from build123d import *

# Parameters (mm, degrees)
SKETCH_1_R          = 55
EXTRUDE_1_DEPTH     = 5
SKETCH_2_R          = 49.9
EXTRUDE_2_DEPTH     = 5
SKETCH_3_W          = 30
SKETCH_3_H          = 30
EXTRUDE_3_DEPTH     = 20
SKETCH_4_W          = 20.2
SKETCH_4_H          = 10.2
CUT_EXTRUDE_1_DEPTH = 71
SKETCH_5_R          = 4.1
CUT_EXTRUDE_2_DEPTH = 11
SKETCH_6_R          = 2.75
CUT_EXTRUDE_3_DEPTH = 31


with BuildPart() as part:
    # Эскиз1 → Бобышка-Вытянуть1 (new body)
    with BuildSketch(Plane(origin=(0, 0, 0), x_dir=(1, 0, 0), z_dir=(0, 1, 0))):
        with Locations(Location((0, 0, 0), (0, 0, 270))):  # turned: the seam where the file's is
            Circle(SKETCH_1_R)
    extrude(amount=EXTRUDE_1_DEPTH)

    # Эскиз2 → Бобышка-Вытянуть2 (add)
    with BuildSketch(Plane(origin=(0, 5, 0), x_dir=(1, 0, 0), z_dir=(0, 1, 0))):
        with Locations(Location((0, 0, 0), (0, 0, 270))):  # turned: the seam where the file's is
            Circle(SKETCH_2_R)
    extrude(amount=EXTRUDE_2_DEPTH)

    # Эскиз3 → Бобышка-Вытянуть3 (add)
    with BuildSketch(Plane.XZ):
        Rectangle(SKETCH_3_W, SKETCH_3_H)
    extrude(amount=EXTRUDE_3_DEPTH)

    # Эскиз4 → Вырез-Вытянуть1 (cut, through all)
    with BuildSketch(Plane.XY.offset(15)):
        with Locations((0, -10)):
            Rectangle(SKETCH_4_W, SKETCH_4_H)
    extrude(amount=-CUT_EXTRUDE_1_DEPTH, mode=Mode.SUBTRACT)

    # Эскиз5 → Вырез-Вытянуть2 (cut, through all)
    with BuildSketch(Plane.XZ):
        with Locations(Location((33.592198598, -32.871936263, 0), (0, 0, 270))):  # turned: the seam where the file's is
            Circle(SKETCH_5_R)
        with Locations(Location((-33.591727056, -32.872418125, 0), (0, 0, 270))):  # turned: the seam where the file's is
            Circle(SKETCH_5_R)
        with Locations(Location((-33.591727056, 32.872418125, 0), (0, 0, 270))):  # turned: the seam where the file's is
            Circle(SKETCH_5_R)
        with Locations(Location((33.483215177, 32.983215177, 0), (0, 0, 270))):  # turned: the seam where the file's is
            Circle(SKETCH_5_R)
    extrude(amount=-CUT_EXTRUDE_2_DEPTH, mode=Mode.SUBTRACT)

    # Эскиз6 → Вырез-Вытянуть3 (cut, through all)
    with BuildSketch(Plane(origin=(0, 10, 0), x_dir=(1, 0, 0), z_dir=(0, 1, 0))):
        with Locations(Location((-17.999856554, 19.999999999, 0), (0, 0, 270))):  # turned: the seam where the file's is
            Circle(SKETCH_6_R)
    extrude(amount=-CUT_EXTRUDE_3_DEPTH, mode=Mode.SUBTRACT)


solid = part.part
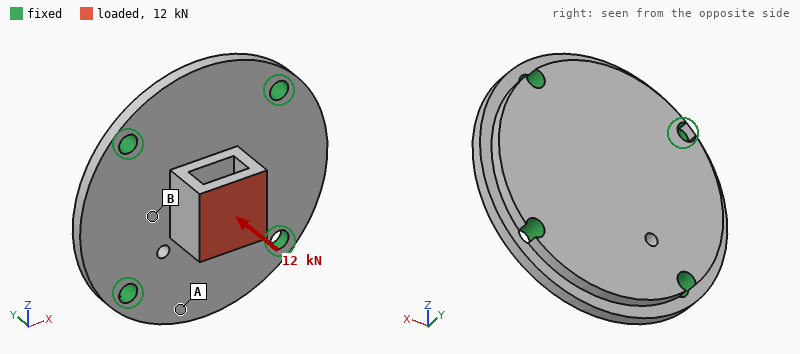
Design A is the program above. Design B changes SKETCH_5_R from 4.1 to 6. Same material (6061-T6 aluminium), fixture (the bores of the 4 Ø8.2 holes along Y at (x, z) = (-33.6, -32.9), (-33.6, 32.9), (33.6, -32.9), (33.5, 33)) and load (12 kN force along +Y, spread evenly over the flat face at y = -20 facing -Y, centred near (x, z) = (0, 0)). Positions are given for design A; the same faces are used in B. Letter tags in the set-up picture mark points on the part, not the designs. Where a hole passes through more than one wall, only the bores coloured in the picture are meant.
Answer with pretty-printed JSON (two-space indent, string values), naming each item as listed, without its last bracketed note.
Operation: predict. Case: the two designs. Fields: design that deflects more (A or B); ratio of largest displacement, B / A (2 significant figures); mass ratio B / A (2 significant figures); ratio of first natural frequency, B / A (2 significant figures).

{
  "design that deflects more": "A",
  "ratio of largest displacement, B / A": "0.90",
  "mass ratio B / A": "0.98",
  "ratio of first natural frequency, B / A": "1.1"
}
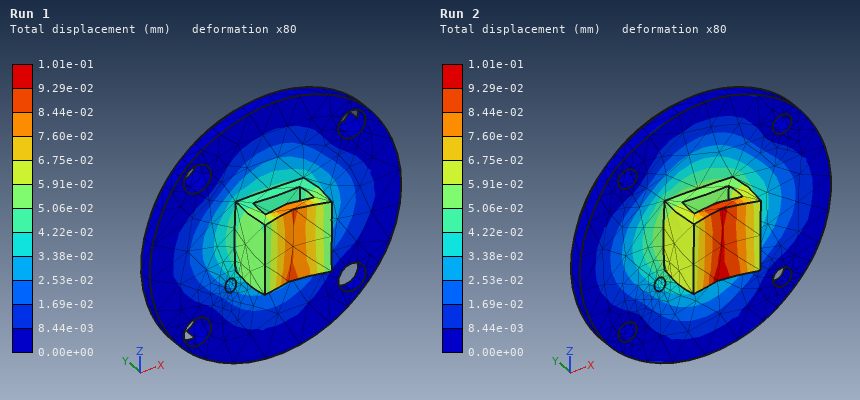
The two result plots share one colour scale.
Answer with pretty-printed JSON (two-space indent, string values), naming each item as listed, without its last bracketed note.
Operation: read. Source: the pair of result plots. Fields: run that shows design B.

{
  "run that shows design B": "Run 1"
}
